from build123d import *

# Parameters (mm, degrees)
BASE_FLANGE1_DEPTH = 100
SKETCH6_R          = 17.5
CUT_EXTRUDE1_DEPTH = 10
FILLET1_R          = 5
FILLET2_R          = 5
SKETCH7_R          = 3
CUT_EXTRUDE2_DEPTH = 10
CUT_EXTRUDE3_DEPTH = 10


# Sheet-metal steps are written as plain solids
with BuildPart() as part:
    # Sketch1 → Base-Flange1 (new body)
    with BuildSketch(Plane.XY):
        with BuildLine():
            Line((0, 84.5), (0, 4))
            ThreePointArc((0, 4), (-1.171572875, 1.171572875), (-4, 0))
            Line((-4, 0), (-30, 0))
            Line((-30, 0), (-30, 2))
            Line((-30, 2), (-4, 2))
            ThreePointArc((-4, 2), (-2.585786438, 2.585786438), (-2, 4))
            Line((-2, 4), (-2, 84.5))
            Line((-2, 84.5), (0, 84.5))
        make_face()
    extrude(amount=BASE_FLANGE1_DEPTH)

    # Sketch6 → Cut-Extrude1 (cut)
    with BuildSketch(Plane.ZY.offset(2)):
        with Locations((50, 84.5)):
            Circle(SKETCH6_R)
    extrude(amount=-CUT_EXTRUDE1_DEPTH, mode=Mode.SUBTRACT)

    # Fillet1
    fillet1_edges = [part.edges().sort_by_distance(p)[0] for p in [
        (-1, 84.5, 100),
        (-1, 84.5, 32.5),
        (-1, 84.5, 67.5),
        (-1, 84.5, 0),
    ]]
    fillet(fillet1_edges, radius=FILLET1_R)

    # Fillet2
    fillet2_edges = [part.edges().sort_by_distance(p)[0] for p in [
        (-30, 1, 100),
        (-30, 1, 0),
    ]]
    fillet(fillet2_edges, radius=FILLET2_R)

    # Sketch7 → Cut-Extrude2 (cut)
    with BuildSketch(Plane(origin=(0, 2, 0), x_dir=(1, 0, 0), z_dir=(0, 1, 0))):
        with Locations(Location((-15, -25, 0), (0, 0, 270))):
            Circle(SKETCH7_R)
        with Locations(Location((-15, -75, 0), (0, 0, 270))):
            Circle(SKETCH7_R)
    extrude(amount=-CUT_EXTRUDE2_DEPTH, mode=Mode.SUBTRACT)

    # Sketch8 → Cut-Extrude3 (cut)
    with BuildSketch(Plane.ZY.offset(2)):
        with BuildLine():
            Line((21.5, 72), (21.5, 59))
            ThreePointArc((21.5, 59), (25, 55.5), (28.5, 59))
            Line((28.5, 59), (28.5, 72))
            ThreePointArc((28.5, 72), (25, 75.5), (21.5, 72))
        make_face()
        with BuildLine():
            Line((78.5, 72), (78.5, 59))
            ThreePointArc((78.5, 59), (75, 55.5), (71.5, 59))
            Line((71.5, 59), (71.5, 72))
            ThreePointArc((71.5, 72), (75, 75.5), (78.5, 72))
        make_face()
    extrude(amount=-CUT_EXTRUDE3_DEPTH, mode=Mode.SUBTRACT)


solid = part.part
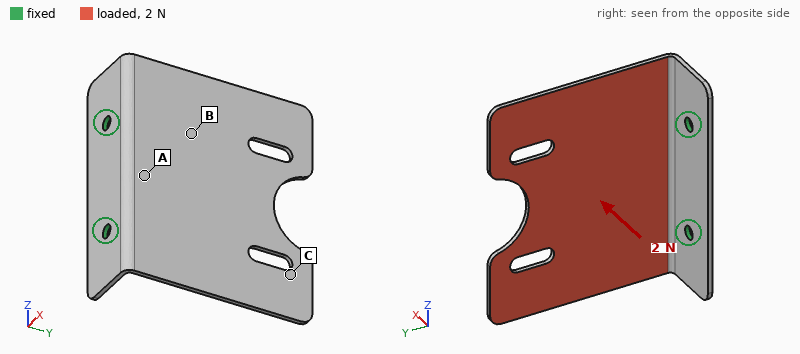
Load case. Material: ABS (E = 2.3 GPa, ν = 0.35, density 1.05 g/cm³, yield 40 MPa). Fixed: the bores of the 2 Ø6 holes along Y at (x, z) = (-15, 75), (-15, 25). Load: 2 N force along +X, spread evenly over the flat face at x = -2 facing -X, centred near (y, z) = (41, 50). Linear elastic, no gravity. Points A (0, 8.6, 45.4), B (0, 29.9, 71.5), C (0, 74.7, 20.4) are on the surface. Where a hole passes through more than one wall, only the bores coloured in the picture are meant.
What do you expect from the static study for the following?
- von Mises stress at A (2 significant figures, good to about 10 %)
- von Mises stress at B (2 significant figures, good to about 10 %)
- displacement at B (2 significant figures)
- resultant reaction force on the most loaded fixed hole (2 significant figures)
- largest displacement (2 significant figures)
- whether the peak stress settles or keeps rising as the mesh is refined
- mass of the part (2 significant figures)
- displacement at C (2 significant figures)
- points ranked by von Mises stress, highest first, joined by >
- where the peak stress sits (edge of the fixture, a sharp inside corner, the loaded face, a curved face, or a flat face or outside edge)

0.91 MPa
0.42 MPa
0.36 mm
1.0 N
1.4 mm
keeps rising
22 g
1.2 mm
A > B > C
edge of the fixture
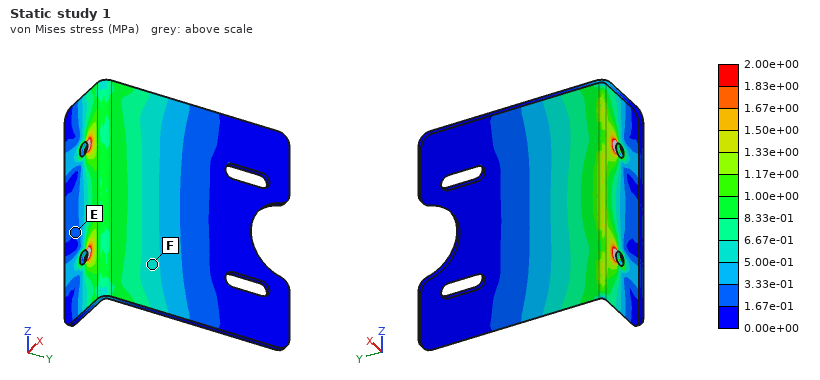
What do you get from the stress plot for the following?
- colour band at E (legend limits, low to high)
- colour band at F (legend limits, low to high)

1.67e-01 to 3.33e-01 MPa
5.00e-01 to 6.67e-01 MPa
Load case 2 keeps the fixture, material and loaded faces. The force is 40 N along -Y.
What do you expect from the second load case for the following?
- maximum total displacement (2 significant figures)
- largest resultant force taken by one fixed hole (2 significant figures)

1.4 mm
20 N
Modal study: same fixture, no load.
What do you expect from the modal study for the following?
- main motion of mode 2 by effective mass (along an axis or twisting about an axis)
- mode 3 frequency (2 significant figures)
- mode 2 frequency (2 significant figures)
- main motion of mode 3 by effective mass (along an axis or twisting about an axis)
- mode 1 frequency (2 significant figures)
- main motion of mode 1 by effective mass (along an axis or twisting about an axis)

twisting about Y
290 Hz
130 Hz
along Z
63 Hz
along X
